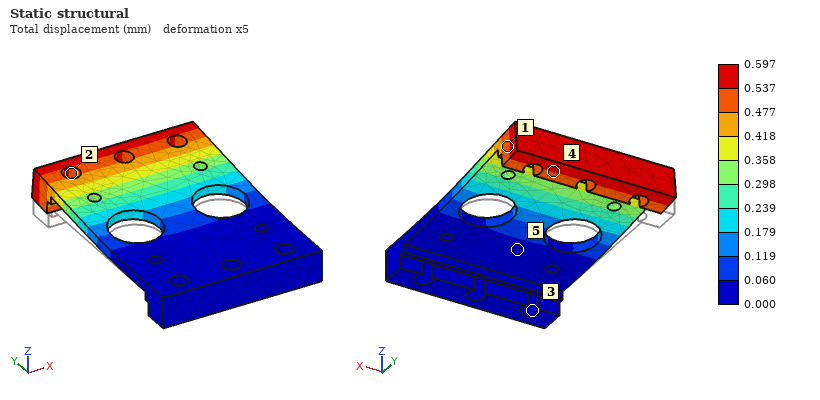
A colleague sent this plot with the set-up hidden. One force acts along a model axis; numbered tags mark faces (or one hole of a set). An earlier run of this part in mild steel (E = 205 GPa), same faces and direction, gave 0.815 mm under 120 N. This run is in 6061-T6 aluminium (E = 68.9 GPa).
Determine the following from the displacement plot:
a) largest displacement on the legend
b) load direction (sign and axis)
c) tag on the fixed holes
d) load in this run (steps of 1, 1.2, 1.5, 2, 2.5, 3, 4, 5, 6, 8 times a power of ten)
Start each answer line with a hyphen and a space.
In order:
- 0.597 mm
- +Z
- 3
- 30 N
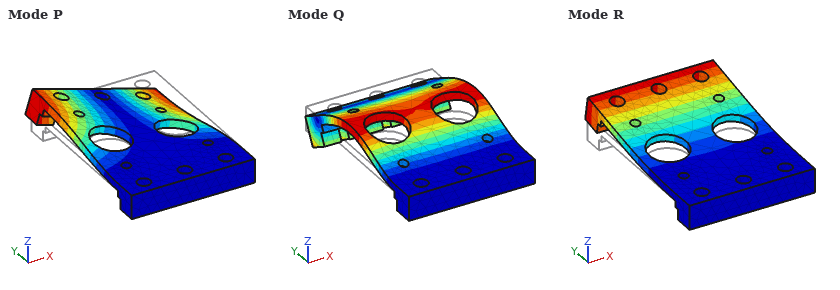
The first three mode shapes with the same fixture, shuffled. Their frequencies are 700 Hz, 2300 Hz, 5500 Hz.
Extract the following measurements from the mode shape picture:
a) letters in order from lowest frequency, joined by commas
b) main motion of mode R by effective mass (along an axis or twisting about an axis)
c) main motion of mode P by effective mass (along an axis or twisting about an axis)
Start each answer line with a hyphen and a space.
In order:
- R, P, Q
- along Z
- twisting about Y
